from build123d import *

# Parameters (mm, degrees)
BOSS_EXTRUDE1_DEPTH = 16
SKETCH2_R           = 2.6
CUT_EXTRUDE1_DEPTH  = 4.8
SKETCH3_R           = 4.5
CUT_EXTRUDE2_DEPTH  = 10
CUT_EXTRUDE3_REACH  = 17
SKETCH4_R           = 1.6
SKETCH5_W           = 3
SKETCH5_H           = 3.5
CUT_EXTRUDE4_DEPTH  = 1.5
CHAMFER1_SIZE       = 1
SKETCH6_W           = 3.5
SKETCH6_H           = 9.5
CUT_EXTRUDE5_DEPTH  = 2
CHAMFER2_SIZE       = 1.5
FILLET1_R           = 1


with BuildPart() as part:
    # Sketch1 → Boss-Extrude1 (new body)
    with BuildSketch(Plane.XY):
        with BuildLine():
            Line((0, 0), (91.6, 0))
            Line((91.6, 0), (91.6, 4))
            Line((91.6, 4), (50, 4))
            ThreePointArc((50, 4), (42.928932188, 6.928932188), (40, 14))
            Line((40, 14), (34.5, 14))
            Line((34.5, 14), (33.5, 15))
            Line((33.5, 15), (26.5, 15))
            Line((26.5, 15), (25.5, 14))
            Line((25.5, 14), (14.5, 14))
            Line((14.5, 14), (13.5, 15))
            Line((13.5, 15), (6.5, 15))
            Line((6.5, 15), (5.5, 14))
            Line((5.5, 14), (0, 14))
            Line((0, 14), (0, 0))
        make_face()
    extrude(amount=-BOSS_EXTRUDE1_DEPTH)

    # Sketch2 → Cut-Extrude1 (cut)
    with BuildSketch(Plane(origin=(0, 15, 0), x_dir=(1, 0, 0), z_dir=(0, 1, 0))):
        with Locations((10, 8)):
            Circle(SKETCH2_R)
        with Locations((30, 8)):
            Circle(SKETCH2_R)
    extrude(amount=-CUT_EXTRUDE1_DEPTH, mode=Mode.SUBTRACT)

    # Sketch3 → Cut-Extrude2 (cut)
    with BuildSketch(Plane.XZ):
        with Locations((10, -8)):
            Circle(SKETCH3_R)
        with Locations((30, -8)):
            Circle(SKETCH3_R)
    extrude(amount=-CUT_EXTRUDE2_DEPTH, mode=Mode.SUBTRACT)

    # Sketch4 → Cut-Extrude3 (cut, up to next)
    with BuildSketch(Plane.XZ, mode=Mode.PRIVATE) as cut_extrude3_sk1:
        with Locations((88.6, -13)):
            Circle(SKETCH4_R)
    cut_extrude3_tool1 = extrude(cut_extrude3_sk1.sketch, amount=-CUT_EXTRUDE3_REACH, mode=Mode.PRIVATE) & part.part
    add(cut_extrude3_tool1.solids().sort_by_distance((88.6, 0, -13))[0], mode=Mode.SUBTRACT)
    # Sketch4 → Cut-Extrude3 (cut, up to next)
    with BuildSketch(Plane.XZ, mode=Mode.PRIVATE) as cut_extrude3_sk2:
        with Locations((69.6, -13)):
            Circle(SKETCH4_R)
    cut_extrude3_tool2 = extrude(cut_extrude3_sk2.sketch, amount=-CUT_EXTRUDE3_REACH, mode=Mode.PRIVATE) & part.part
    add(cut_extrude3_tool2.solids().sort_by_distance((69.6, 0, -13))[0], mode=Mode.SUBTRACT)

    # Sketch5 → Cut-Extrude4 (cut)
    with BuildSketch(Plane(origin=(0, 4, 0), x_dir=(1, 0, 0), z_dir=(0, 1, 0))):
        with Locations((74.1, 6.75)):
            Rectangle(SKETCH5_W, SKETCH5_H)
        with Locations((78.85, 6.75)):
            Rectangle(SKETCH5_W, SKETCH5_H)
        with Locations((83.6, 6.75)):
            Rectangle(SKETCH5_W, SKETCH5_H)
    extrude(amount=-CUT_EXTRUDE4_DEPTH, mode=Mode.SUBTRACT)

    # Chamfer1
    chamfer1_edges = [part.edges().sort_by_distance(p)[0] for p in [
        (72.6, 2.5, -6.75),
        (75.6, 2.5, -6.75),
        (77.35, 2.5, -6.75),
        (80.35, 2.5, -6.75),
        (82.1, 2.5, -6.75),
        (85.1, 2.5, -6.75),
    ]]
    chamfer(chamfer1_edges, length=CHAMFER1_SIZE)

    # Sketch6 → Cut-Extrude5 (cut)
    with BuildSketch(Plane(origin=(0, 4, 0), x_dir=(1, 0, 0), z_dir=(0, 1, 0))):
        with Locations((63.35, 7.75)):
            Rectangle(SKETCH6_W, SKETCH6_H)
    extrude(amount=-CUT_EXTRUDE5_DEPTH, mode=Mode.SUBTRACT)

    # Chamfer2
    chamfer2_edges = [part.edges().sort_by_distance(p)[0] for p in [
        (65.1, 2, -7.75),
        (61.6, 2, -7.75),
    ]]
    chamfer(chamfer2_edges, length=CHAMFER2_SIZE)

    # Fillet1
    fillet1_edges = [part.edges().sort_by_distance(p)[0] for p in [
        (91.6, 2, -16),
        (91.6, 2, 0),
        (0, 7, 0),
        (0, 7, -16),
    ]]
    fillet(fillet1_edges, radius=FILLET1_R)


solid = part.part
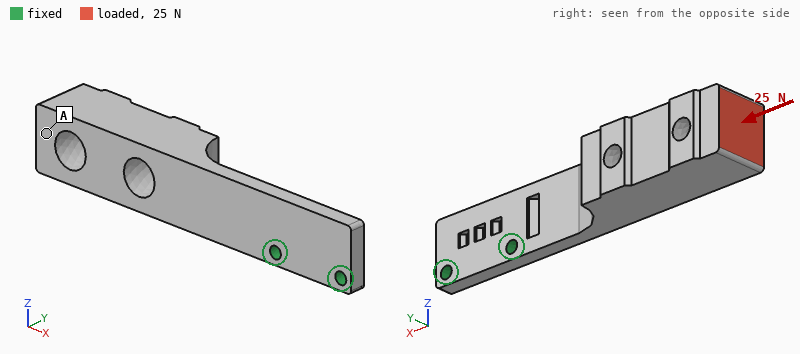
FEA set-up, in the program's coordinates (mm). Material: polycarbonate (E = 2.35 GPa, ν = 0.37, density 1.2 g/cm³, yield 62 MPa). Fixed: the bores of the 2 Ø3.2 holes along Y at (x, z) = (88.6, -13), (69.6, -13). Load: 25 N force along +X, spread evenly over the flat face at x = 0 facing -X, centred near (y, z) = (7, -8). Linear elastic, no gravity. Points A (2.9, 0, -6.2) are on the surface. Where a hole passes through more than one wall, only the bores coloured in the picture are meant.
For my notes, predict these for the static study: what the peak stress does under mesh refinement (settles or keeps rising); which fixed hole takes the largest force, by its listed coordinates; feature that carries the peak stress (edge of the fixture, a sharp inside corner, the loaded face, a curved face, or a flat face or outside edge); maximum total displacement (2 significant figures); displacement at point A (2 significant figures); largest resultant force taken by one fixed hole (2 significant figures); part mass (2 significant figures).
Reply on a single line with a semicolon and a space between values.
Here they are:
keeps rising; (69.6, -13); edge of the fixture; 1.1 mm; 1.0 mm; 20 N; 13 g
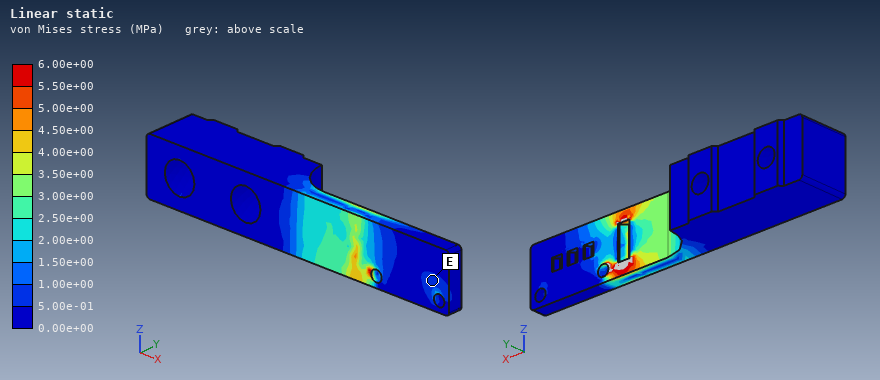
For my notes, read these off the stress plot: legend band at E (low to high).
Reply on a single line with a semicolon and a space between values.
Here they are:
5.00e-01 to 1.00e+00 MPa
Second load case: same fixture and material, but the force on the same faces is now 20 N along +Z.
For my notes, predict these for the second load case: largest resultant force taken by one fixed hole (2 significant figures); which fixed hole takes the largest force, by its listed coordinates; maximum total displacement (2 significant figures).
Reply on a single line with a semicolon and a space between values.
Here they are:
97 N; (69.6, -13); 0.94 mm
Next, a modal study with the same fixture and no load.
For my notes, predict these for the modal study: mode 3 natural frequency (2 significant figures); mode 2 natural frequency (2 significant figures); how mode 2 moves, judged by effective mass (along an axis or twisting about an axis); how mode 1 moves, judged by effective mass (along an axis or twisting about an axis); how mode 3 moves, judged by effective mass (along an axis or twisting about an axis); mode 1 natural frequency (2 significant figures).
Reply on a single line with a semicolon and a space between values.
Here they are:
750 Hz; 340 Hz; along Z; along Y; twisting about X; 100 Hz
